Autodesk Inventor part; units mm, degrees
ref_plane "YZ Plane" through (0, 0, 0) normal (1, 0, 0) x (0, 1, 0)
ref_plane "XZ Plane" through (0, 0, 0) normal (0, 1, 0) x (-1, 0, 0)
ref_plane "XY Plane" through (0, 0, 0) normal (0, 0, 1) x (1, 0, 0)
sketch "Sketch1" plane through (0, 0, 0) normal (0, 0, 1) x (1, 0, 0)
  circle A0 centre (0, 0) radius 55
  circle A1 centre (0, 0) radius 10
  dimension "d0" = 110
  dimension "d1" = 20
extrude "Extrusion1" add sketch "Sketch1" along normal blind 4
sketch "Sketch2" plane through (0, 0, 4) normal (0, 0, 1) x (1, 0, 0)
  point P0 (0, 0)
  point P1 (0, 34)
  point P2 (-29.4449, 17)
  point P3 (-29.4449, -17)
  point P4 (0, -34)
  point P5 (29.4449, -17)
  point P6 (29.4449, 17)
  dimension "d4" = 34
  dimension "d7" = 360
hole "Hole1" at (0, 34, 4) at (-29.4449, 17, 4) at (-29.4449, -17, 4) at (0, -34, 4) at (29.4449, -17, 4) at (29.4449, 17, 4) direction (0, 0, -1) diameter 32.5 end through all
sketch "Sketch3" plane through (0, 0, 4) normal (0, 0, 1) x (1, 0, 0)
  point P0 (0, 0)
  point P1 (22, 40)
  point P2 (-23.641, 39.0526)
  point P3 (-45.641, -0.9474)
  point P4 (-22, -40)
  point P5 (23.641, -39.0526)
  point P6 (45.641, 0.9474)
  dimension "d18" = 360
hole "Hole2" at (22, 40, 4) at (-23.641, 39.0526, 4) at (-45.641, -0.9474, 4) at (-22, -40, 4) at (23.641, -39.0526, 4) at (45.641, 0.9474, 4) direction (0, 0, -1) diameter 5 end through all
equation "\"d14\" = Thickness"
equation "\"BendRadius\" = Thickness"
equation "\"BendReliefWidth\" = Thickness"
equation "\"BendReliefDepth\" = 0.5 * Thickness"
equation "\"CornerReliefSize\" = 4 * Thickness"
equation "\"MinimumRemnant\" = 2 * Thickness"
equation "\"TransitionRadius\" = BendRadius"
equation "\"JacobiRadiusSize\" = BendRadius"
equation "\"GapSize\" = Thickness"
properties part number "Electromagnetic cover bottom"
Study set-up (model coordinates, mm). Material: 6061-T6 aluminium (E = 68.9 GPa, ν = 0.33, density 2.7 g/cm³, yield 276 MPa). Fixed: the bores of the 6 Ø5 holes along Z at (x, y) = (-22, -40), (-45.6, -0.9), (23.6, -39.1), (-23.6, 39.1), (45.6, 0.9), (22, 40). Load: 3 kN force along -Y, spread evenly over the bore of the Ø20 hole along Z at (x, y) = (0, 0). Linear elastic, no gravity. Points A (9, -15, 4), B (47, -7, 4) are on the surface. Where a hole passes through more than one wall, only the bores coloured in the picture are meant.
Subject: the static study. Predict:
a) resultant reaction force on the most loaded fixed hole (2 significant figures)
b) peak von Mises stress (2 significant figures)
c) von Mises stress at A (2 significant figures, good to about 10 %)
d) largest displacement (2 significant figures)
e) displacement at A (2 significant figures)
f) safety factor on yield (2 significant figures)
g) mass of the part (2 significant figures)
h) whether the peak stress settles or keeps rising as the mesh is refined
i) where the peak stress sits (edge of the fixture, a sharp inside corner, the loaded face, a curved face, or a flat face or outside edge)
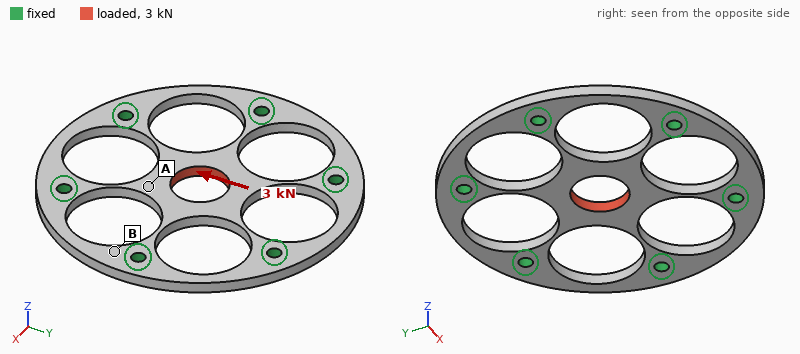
810 N
150 MPa
24 MPa
32 µm
29 µm
1.8
44 g
settles
a curved face
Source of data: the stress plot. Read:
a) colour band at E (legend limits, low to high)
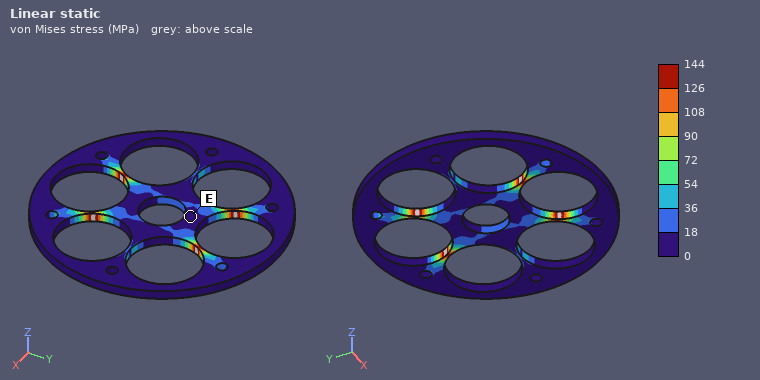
0 to 18 MPa
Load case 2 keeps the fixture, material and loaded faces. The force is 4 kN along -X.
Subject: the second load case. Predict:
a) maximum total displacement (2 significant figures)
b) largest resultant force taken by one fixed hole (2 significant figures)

42 µm
1.2 kN
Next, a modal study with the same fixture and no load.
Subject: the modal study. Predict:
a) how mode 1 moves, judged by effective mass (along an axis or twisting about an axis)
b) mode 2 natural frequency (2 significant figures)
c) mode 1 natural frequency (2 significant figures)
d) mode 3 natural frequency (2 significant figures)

along Z
6500 Hz
3100 Hz
6500 Hz
